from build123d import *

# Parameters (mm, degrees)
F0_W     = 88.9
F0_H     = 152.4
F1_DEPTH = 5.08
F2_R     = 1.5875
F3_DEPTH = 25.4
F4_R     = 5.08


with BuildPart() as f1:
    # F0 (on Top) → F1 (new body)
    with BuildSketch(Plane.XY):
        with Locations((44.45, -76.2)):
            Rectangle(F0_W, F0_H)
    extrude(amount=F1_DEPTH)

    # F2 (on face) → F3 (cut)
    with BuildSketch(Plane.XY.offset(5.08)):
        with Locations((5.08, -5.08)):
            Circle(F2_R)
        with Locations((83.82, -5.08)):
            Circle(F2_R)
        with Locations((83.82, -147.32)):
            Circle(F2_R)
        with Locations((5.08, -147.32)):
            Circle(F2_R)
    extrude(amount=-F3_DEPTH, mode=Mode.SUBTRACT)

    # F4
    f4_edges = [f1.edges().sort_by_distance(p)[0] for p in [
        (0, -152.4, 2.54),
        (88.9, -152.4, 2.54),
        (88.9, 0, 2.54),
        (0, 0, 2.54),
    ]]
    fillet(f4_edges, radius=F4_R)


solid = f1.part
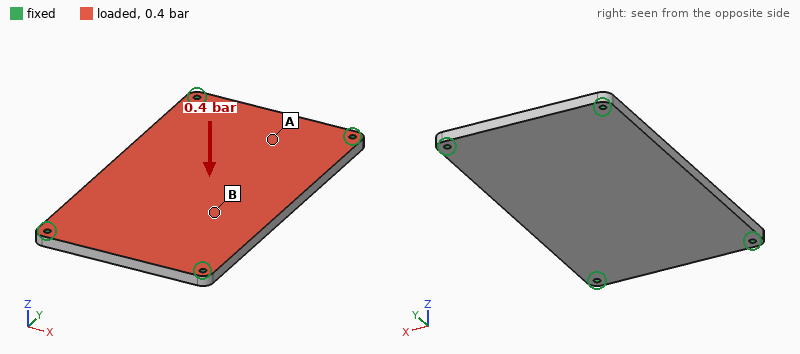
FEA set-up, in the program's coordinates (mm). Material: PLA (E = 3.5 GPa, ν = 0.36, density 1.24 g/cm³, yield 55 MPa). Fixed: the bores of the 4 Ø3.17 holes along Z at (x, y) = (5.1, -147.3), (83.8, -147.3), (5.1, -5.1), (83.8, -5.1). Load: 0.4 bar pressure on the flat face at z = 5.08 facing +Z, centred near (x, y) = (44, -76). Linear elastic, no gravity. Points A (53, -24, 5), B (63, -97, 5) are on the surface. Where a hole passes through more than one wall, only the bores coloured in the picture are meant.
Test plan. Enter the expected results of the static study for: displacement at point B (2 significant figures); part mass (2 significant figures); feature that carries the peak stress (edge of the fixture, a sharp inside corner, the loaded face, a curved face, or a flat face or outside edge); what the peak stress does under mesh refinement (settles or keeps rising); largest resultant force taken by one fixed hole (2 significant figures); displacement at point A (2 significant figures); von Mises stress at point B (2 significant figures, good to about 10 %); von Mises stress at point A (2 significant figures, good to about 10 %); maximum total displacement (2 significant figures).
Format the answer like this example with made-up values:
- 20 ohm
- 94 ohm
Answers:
- 1.6 mm
- 85 g
- edge of the fixture
- keeps rising
- 130 N
- 0.76 mm
- 7.9 MPa
- 3.8 MPa
- 1.9 mm
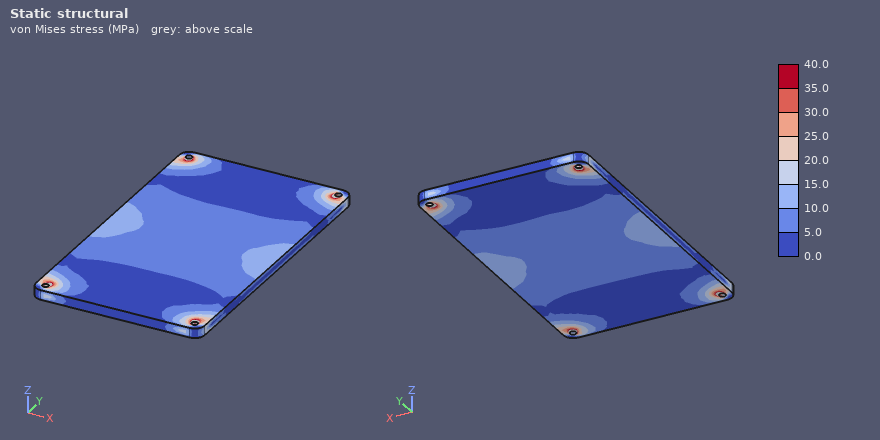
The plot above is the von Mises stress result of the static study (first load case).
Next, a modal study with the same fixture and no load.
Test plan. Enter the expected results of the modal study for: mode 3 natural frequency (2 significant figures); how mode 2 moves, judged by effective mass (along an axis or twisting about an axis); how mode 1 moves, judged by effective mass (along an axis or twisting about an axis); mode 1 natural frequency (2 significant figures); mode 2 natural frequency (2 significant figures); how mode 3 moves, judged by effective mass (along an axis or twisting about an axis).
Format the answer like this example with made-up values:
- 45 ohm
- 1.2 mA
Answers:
- 910 Hz
- twisting about Y
- along Z
- 330 Hz
- 590 Hz
- twisting about X
